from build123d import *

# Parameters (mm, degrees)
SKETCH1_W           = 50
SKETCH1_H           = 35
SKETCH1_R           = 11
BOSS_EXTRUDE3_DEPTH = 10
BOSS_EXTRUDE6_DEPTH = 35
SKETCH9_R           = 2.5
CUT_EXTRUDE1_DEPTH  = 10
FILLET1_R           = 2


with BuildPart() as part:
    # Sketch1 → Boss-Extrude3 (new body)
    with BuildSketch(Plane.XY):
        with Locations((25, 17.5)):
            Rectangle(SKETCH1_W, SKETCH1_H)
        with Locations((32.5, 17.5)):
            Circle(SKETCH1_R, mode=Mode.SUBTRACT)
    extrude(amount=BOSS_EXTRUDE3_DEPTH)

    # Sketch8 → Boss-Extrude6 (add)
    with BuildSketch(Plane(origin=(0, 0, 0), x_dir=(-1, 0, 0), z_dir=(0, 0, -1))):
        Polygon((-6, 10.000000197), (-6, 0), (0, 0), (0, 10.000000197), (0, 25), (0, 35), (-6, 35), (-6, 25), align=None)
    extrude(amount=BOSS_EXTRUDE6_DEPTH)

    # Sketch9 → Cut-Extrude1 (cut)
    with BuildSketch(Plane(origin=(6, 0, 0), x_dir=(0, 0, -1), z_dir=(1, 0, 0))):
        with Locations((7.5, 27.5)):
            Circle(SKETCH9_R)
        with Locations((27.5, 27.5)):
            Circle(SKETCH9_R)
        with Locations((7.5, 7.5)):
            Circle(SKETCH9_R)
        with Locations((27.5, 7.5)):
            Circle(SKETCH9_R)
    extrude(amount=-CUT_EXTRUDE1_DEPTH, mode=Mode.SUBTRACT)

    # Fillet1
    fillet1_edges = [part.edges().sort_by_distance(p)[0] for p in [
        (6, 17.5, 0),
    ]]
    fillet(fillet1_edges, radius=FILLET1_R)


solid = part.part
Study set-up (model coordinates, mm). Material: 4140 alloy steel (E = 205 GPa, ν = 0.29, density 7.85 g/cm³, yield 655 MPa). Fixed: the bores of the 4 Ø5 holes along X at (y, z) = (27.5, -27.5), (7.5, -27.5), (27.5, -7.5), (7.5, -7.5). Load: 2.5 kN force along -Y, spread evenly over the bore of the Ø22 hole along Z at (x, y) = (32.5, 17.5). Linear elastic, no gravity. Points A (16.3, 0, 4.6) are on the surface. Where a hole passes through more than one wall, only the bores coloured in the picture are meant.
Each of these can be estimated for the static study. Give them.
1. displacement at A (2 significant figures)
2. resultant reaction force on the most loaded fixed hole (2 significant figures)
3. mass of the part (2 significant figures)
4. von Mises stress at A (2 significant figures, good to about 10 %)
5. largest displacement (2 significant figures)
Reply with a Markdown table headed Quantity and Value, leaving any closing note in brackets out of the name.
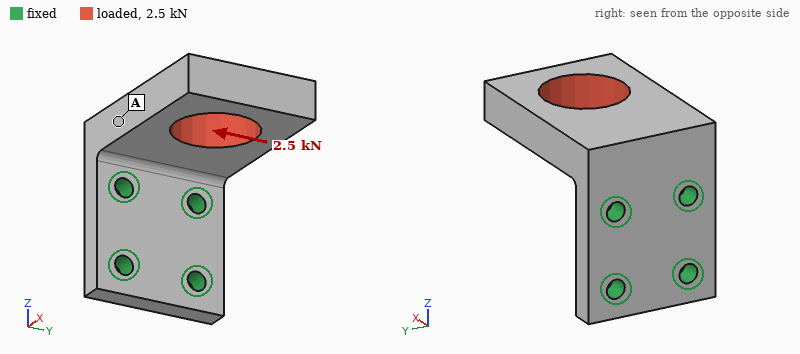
| Quantity | Value |
|---|---|
| displacement at A | 23 µm |
| resultant reaction force on the most loaded fixed hole | 3.5 kN |
| mass of the part | 160 g |
| von Mises stress at A | 38 MPa |
| largest displacement | 66 µm |
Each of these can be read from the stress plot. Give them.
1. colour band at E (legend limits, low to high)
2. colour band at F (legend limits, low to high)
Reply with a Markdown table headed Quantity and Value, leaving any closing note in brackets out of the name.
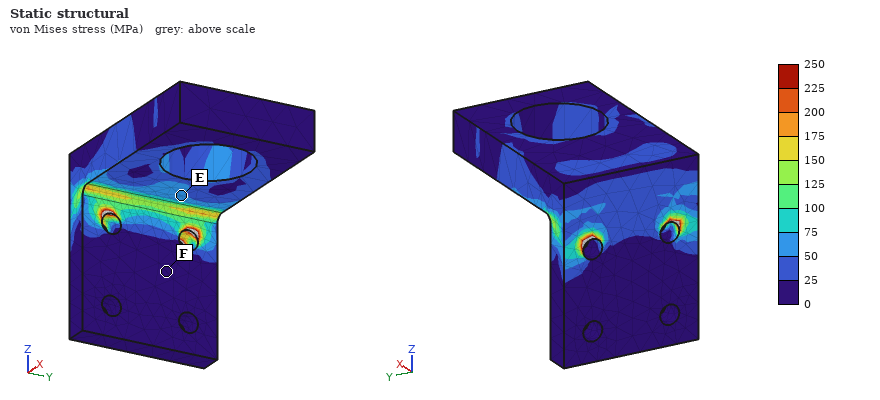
| Quantity | Value |
|---|---|
| colour band at E | 50 to 75 MPa |
| colour band at F | 0 to 25 MPa |
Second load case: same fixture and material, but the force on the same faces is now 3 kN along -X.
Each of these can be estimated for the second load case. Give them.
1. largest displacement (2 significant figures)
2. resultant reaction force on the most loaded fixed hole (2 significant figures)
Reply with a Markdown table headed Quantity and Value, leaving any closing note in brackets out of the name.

| Quantity | Value |
|---|---|
| largest displacement | 78 µm |
| resultant reaction force on the most loaded fixed hole | 1.7 kN |
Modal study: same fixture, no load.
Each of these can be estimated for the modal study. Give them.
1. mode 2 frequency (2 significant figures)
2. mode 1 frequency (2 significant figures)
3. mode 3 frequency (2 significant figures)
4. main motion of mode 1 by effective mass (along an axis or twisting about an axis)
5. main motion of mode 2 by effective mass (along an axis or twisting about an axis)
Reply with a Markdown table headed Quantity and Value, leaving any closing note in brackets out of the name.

| Quantity | Value |
|---|---|
| mode 2 frequency | 4300 Hz |
| mode 1 frequency | 2000 Hz |
| mode 3 frequency | 7500 Hz |
| main motion of mode 1 by effective mass | along Z |
| main motion of mode 2 by effective mass | along Y |
